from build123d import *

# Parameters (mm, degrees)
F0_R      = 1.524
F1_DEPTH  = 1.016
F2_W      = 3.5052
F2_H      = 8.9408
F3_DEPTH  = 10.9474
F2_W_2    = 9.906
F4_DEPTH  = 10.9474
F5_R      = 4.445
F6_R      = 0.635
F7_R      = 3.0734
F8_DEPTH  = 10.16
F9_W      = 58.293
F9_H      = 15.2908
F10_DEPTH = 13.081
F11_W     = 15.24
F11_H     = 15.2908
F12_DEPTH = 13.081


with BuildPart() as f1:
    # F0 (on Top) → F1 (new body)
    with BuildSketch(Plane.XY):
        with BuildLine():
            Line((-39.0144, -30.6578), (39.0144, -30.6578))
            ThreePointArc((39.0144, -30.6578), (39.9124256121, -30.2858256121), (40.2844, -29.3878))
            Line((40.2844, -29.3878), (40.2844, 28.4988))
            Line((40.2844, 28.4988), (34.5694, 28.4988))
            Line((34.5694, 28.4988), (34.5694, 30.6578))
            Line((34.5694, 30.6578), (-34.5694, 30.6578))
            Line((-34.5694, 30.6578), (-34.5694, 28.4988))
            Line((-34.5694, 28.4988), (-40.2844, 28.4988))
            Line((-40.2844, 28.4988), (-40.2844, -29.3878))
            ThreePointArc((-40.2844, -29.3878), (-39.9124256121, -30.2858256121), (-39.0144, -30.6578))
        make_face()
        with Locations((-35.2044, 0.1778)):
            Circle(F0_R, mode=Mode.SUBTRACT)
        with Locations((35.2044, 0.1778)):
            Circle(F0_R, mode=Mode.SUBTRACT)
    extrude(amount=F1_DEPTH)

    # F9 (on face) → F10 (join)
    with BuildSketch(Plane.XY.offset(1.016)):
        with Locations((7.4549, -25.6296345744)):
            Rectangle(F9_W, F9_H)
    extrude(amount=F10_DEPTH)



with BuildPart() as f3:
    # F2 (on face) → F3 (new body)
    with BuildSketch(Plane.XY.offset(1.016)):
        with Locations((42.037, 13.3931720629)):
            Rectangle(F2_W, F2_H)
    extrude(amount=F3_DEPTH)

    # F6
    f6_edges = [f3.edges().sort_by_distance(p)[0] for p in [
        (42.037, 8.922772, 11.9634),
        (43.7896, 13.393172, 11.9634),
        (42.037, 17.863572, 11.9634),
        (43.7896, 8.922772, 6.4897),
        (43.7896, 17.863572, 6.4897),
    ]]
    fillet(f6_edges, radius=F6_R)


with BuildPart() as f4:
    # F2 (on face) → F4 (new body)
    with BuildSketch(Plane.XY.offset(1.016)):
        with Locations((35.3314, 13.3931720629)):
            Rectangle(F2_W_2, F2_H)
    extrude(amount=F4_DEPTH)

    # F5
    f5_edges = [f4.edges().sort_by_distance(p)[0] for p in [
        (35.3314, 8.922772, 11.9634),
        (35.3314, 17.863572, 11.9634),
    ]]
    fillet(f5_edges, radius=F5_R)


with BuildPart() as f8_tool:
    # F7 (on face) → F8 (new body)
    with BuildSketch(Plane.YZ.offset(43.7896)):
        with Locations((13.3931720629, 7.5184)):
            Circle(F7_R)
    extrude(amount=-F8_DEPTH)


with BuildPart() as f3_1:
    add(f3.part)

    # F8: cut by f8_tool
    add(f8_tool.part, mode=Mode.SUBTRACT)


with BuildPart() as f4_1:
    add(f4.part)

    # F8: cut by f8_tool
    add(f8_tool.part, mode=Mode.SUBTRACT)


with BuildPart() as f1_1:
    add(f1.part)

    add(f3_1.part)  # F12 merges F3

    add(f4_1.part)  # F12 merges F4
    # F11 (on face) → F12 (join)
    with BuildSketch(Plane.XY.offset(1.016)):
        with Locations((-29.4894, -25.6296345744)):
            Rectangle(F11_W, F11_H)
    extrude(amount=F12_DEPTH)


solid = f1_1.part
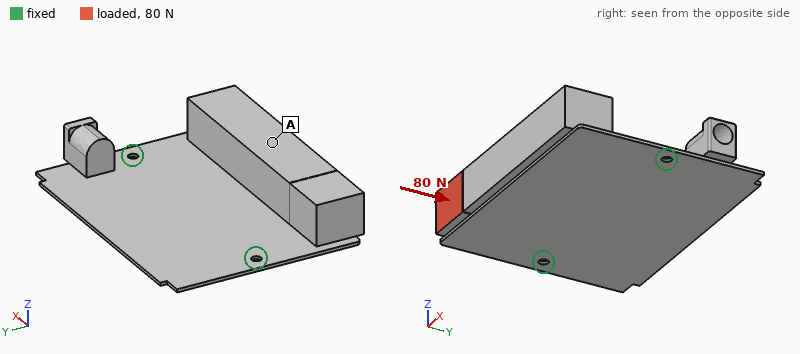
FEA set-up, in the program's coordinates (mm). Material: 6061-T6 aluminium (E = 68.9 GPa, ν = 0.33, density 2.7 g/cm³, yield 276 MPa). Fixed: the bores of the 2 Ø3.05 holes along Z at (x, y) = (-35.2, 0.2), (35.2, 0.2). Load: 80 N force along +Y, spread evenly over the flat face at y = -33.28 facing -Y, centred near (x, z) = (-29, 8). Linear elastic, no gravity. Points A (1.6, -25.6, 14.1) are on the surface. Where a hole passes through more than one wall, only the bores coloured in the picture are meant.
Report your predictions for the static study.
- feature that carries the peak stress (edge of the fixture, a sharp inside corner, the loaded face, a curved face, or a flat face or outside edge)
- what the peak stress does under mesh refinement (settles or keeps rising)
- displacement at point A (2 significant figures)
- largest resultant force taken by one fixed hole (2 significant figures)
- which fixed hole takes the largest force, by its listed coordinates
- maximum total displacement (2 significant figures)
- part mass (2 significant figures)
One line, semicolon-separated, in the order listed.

edge of the fixture; keeps rising; 0.57 mm; 73 N; (-35.2, 0.2); 0.74 mm; 56 g
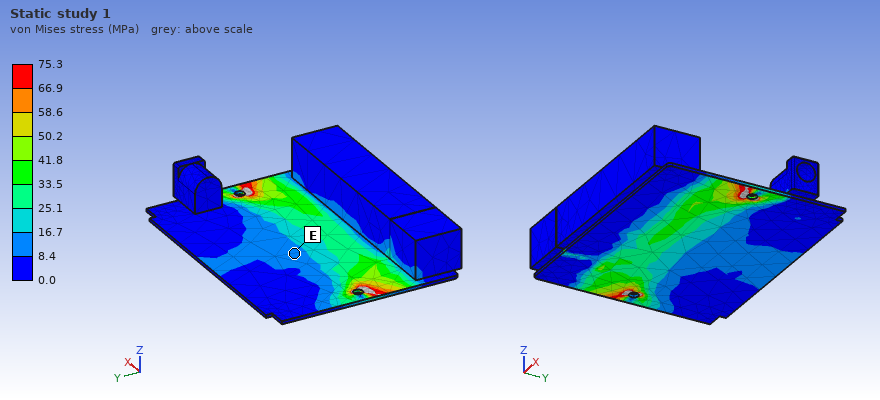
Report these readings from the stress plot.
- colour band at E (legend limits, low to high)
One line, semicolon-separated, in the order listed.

8.4 to 16.7 MPa
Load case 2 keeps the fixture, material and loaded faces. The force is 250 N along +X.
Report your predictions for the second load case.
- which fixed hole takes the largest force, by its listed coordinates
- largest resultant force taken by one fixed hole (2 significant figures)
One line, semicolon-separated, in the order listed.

(35.2, 0.2); 190 N
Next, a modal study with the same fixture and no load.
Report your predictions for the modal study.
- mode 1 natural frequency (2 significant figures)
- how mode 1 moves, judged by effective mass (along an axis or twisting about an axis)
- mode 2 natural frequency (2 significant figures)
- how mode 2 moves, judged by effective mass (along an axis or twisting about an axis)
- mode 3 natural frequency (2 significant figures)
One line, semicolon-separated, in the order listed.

170 Hz; along Z; 630 Hz; along Z; 760 Hz
